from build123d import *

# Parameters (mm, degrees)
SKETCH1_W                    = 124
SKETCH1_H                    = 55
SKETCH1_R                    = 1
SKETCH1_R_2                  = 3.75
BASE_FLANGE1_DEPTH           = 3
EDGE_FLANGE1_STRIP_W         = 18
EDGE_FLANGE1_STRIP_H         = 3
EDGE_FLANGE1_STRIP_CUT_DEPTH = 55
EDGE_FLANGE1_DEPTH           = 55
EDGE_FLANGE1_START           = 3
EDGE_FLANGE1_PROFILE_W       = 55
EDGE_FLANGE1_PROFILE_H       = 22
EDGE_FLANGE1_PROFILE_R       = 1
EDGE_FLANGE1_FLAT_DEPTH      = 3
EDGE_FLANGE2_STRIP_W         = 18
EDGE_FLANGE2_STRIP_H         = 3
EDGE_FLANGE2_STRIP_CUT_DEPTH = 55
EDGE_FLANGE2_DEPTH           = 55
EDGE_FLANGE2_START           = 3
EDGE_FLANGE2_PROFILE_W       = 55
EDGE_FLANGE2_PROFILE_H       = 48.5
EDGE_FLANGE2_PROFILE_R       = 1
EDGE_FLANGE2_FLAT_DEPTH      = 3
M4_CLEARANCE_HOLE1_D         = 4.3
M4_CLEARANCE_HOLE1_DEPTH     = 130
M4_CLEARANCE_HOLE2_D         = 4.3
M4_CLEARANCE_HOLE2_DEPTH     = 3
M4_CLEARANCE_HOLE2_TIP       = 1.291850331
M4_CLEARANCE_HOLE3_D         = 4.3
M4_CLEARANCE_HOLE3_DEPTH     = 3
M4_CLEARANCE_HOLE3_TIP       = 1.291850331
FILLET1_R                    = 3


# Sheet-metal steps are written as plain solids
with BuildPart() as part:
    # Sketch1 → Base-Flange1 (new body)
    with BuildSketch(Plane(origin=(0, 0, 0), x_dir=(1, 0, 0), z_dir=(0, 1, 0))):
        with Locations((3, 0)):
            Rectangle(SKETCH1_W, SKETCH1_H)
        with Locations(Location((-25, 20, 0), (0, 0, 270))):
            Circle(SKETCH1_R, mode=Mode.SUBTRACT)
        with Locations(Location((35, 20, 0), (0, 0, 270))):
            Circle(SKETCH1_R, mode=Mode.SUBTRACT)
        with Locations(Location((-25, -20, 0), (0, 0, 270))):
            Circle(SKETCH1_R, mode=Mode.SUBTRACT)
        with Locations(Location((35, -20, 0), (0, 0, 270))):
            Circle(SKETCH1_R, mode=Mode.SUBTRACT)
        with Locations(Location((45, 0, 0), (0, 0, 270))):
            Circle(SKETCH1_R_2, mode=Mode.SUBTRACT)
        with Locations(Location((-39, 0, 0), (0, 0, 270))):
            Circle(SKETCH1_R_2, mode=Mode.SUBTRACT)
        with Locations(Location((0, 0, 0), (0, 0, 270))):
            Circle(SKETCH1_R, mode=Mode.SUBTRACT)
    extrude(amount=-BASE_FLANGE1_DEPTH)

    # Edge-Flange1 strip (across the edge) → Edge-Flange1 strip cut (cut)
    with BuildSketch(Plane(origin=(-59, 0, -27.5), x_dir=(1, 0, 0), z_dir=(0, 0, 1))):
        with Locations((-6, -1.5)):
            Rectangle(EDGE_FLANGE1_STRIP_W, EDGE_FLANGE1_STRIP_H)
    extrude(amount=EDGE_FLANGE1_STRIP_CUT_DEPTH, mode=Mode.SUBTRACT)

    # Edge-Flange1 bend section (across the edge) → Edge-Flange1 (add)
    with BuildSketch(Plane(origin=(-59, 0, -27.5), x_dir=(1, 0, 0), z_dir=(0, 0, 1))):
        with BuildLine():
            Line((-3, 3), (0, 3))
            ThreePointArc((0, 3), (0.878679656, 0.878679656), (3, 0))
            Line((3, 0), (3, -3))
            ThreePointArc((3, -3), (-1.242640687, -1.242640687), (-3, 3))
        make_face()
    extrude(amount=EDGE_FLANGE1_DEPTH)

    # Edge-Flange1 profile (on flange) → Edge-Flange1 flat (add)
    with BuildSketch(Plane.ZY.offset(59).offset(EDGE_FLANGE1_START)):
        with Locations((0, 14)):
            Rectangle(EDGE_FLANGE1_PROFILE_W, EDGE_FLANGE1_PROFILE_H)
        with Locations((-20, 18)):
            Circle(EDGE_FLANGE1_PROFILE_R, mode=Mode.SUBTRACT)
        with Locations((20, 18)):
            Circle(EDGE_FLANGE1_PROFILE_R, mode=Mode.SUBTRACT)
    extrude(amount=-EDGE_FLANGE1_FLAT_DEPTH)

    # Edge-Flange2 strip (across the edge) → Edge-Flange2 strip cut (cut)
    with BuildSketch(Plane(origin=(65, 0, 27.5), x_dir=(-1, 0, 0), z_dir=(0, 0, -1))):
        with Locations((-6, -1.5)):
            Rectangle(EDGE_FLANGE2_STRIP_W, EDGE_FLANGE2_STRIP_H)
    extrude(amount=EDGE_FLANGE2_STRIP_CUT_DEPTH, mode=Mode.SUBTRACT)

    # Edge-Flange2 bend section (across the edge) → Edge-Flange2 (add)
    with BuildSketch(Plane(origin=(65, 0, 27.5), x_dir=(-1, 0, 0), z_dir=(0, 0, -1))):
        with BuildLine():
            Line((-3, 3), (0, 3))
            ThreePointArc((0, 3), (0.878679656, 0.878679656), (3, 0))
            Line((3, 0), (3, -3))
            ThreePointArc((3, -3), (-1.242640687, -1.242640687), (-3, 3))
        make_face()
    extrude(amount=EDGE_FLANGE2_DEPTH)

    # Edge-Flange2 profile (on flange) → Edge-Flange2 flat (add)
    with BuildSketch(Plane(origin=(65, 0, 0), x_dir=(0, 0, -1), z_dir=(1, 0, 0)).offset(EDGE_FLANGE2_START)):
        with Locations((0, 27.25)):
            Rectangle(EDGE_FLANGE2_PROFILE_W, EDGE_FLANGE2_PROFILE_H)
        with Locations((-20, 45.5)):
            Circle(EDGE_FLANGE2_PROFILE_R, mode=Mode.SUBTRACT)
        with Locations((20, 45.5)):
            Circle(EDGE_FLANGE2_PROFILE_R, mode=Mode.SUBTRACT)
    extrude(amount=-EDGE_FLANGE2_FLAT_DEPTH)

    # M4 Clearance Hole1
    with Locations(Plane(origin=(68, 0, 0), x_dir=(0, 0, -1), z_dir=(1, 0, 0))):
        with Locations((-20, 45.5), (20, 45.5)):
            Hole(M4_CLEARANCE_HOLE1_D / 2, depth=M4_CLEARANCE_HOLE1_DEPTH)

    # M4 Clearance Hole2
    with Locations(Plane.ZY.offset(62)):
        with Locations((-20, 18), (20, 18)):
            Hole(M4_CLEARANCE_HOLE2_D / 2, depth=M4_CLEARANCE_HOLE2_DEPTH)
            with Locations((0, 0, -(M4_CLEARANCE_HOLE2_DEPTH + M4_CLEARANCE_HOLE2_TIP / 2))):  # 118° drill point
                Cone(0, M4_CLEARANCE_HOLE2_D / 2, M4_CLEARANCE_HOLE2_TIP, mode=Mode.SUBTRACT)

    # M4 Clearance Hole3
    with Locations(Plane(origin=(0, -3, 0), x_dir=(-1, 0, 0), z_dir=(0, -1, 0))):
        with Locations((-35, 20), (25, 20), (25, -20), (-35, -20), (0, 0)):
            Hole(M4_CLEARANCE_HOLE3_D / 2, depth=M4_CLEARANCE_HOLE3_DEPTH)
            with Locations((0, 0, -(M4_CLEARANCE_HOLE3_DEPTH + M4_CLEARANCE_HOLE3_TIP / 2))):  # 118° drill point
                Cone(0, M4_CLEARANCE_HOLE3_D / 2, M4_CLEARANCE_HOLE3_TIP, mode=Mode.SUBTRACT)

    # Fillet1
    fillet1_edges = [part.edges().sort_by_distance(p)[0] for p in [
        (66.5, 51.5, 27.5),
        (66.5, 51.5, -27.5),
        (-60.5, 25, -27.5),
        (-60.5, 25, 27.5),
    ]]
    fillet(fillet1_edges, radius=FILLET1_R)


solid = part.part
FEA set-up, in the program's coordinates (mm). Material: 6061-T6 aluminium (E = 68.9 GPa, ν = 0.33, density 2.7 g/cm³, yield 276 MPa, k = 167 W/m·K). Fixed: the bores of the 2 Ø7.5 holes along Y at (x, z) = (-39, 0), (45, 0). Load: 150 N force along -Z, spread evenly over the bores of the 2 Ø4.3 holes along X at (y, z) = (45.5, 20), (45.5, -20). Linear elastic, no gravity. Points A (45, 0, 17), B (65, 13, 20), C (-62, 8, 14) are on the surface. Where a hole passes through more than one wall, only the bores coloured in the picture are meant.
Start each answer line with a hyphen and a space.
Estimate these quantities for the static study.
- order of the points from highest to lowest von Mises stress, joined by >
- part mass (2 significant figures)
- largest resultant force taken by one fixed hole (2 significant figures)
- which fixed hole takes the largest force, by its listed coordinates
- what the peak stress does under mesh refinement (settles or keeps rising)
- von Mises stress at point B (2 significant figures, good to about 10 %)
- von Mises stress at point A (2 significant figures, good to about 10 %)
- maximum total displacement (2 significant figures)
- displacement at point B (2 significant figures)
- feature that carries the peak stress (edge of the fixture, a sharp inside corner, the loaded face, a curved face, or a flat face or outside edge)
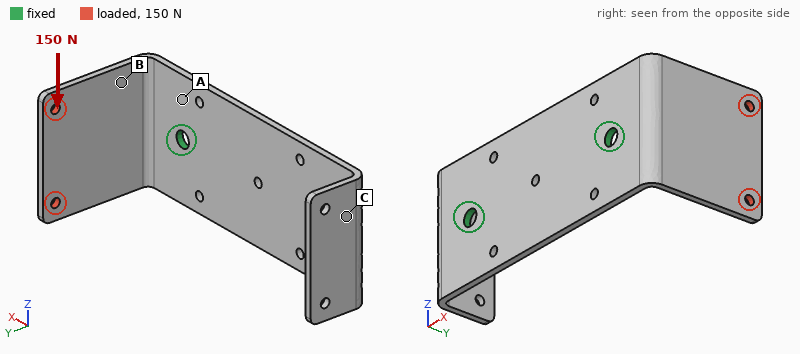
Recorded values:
- A > B > C
- 88 g
- 180 N
- (45, 0)
- keeps rising
- 20 MPa
- 38 MPa
- 0.55 mm
- 0.24 mm
- edge of the fixture
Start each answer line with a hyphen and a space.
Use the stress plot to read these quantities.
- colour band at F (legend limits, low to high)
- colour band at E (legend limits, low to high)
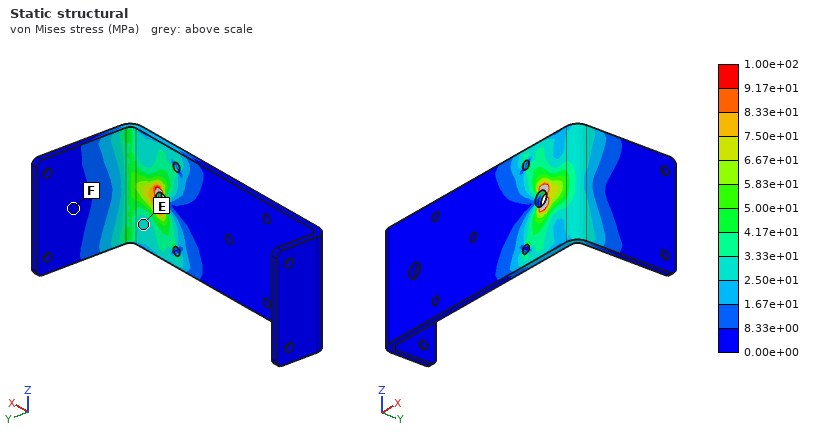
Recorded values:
- 0.00e+00 to 8.33e+00 MPa
- 2.50e+01 to 3.33e+01 MPa
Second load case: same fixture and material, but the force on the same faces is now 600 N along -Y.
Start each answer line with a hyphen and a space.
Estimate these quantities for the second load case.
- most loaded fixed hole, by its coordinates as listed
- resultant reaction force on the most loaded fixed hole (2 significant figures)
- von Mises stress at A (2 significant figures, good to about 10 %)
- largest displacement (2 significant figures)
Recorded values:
- (45, 0)
- 620 N
- 56 MPa
- 0.91 mm
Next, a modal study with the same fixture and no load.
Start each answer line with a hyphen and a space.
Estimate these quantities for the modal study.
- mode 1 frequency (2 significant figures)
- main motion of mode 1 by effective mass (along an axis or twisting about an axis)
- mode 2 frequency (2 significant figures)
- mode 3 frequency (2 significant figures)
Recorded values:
- 550 Hz
- along X
- 820 Hz
- 1500 Hz
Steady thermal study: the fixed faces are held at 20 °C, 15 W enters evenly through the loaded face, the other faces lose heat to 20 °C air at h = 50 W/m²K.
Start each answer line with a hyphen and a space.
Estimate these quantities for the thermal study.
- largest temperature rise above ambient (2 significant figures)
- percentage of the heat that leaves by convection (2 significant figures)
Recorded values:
- 32 K
- 46 %
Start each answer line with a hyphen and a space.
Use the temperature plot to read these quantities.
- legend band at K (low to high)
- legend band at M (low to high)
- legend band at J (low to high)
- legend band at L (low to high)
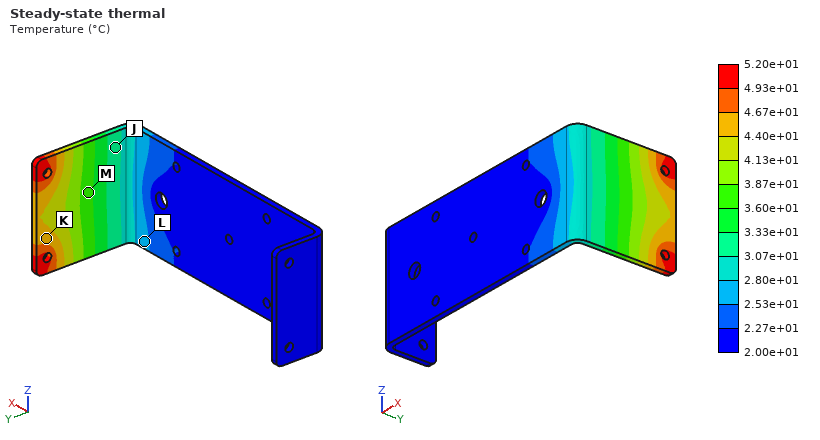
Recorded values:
- 4.40e+01 to 4.67e+01 °C
- 3.60e+01 to 3.87e+01 °C
- 3.07e+01 to 3.33e+01 °C
- 2.53e+01 to 2.80e+01 °C
